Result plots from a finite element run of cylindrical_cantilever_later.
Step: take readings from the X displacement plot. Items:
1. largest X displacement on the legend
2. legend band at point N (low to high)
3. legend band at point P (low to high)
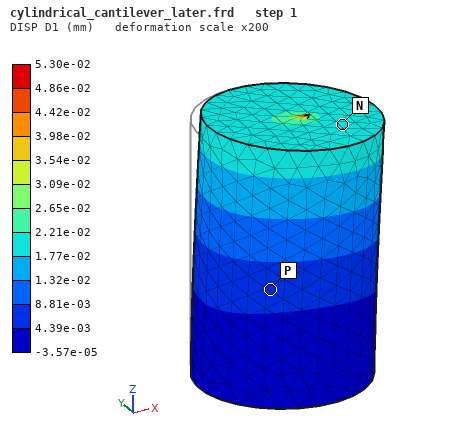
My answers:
5.30e-02 mm
1.77e-02 to 2.21e-02 mm
4.39e-03 to 8.81e-03 mm
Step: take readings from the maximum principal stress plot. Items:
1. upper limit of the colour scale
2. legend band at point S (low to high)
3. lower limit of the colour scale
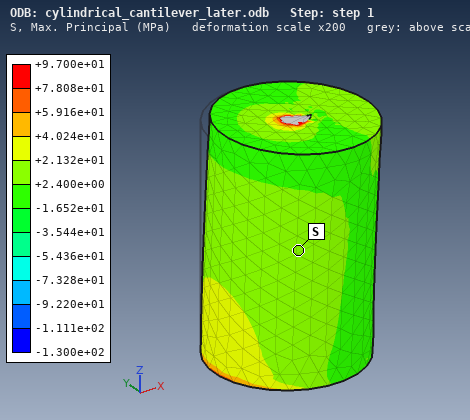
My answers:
+9.700e+01 MPa
+2.400e+00 to +2.132e+01 MPa
-1.300e+02 MPa
